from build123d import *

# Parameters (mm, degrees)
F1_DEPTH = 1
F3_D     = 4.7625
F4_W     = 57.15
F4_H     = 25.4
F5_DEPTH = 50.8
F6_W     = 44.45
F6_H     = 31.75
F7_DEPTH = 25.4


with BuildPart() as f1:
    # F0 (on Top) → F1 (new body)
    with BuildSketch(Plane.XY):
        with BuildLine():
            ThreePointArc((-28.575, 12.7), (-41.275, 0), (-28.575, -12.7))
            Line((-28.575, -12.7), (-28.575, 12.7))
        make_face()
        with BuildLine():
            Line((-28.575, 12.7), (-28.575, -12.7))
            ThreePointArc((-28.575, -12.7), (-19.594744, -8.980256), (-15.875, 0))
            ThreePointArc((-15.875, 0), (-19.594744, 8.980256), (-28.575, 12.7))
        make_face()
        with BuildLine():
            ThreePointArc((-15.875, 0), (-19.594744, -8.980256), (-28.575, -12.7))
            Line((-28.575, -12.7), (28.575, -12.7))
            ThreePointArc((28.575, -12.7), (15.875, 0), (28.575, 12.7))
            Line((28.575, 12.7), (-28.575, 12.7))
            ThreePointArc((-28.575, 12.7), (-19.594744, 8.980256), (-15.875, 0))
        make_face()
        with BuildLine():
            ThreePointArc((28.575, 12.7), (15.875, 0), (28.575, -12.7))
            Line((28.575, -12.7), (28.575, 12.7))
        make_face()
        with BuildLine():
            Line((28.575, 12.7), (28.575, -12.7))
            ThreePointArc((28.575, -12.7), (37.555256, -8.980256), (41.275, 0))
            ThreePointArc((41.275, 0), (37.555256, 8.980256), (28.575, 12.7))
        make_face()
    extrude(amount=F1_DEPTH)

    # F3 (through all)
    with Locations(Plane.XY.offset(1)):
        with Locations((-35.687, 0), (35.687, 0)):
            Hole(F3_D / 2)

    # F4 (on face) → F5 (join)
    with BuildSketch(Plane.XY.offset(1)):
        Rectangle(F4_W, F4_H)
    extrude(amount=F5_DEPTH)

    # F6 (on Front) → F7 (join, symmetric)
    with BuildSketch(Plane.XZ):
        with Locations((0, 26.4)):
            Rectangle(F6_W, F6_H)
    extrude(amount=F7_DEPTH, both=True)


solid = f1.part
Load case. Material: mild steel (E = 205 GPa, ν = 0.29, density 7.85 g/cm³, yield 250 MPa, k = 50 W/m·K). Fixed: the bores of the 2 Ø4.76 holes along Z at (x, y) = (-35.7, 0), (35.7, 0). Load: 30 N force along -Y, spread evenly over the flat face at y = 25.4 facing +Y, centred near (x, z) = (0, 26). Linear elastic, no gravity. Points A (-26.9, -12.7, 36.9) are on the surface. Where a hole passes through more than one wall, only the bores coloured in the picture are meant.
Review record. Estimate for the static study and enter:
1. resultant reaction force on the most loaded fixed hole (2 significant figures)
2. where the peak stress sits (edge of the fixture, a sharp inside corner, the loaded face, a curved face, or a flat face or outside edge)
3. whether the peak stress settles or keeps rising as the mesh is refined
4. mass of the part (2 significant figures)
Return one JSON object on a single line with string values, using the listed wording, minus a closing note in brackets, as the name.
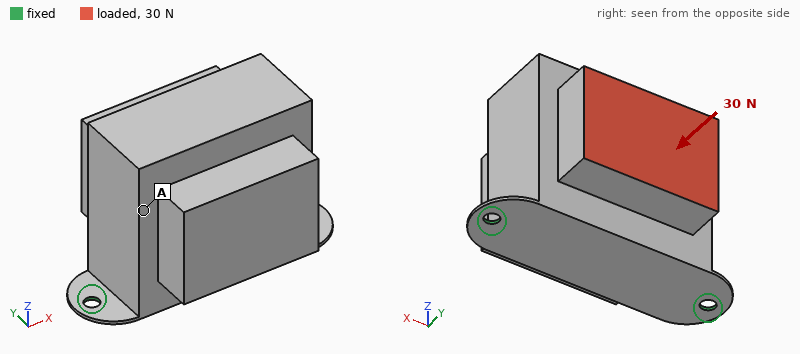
{"resultant reaction force on the most loaded fixed hole": "15 N", "where the peak stress sits": "edge of the fixture", "whether the peak stress settles or keeps rising as the mesh is refined": "keeps rising", "mass of the part": "880 g"}
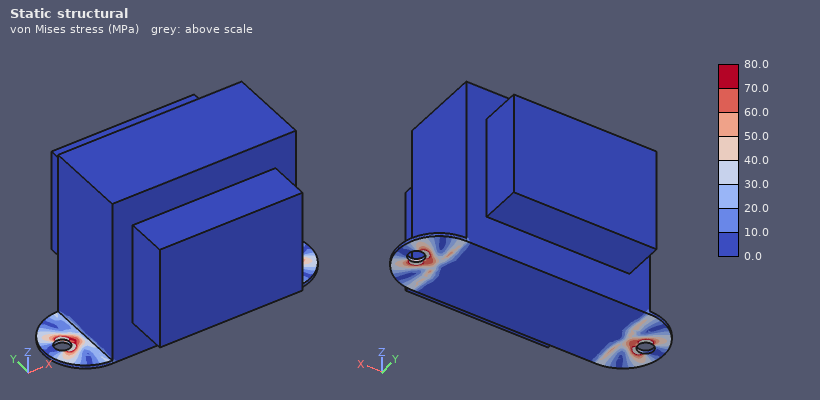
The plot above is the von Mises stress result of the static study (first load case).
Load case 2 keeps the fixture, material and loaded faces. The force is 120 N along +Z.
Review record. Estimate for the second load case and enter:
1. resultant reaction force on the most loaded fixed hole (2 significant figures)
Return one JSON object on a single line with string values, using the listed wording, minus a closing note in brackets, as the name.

{"resultant reaction force on the most loaded fixed hole": "69 N"}
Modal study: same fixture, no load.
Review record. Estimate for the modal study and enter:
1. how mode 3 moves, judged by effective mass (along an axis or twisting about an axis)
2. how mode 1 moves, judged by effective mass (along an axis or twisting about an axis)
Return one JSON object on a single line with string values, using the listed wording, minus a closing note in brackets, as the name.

{"how mode 3 moves, judged by effective mass": "along Z", "how mode 1 moves, judged by effective mass": "along Y"}
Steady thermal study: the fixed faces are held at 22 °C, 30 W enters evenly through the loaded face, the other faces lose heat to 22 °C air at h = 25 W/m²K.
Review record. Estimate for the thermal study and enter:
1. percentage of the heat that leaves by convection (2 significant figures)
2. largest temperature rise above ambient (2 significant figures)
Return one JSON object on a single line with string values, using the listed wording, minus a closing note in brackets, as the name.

{"percentage of the heat that leaves by convection": "63 %", "largest temperature rise above ambient": "62 K"}
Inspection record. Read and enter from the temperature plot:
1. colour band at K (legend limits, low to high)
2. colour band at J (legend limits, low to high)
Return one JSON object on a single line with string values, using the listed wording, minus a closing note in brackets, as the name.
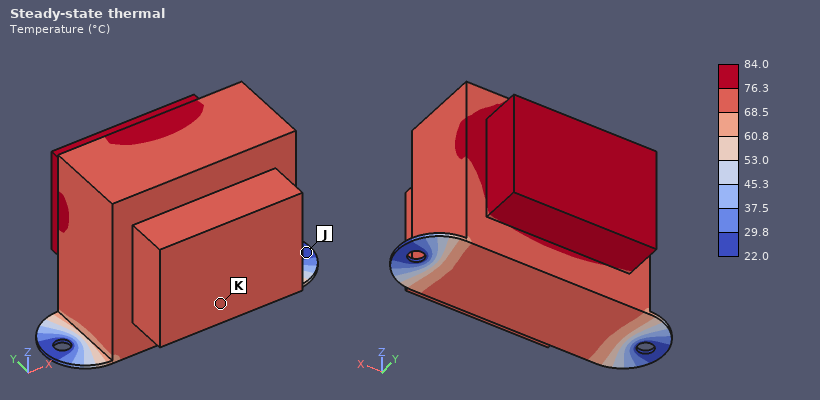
{"colour band at K": "68.5 to 76.3 °C", "colour band at J": "22.0 to 29.8 °C"}
